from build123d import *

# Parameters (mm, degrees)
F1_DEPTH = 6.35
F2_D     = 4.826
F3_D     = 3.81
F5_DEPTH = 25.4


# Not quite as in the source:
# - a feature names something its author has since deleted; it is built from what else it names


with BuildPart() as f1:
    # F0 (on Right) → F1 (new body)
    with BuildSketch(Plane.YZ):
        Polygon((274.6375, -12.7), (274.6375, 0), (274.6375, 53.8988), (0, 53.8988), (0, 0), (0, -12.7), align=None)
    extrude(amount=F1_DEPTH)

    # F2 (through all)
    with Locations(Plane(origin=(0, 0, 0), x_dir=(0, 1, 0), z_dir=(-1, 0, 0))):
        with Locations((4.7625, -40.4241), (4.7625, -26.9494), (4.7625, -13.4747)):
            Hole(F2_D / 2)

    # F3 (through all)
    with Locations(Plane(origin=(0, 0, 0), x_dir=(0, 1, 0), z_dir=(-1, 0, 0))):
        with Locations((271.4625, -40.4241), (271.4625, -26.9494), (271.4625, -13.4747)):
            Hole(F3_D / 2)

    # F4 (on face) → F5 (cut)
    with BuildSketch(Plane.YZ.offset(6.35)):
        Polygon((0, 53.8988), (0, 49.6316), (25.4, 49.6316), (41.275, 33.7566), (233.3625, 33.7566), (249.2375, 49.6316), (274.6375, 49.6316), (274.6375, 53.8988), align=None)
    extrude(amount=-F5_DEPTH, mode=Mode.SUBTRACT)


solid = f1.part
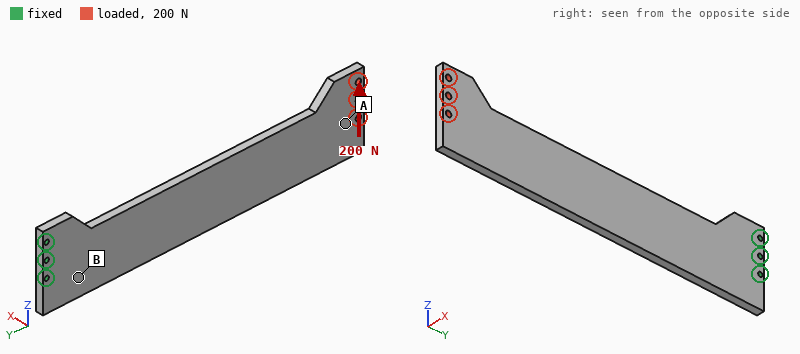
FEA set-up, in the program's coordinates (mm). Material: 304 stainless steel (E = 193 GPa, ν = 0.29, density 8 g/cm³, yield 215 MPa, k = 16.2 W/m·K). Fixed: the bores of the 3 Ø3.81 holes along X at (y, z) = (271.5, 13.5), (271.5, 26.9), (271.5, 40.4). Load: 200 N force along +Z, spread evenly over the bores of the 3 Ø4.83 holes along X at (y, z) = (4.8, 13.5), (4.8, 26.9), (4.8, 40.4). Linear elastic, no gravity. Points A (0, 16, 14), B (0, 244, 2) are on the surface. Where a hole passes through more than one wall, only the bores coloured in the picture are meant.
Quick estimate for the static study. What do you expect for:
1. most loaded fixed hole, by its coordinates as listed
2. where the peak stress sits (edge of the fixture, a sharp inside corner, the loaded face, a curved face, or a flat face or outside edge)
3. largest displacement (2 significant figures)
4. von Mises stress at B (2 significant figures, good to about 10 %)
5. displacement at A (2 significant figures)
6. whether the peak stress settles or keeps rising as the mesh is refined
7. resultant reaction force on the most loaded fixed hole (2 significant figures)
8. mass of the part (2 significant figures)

(271.5, 13.5)
edge of the fixture
0.15 mm
11 MPa
0.13 mm
keeps rising
1.9 kN
700 g
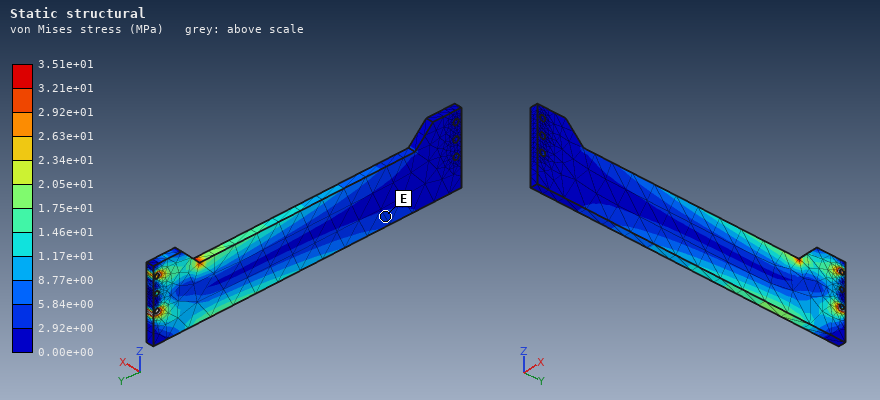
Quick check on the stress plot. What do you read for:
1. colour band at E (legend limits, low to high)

2.92e+00 to 5.84e+00 MPa
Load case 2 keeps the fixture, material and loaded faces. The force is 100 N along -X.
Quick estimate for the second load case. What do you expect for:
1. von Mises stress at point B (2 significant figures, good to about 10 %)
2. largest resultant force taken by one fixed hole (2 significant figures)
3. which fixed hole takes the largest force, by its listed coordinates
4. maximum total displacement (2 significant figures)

63 MPa
260 N
(271.5, 26.9)
3.3 mm
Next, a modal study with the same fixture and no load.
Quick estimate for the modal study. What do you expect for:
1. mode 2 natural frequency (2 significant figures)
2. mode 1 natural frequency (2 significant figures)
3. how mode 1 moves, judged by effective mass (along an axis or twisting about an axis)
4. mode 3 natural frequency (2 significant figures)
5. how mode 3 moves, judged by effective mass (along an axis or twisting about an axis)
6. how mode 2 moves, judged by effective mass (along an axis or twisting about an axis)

410 Hz
66 Hz
along X
430 Hz
along Z
along X
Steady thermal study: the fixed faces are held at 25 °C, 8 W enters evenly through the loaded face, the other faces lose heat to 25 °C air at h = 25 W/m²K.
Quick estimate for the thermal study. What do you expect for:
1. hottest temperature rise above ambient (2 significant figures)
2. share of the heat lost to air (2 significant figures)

65 K
100 %
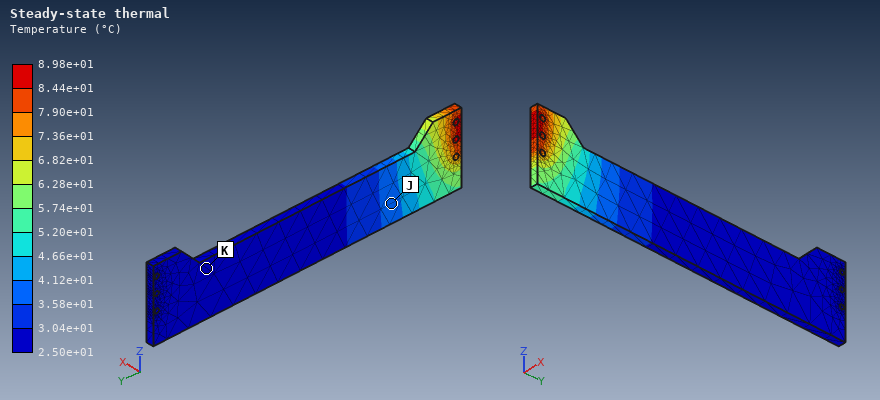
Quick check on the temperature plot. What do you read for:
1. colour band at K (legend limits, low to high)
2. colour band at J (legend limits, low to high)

2.50e+01 to 3.04e+01 °C
3.58e+01 to 4.12e+01 °C
